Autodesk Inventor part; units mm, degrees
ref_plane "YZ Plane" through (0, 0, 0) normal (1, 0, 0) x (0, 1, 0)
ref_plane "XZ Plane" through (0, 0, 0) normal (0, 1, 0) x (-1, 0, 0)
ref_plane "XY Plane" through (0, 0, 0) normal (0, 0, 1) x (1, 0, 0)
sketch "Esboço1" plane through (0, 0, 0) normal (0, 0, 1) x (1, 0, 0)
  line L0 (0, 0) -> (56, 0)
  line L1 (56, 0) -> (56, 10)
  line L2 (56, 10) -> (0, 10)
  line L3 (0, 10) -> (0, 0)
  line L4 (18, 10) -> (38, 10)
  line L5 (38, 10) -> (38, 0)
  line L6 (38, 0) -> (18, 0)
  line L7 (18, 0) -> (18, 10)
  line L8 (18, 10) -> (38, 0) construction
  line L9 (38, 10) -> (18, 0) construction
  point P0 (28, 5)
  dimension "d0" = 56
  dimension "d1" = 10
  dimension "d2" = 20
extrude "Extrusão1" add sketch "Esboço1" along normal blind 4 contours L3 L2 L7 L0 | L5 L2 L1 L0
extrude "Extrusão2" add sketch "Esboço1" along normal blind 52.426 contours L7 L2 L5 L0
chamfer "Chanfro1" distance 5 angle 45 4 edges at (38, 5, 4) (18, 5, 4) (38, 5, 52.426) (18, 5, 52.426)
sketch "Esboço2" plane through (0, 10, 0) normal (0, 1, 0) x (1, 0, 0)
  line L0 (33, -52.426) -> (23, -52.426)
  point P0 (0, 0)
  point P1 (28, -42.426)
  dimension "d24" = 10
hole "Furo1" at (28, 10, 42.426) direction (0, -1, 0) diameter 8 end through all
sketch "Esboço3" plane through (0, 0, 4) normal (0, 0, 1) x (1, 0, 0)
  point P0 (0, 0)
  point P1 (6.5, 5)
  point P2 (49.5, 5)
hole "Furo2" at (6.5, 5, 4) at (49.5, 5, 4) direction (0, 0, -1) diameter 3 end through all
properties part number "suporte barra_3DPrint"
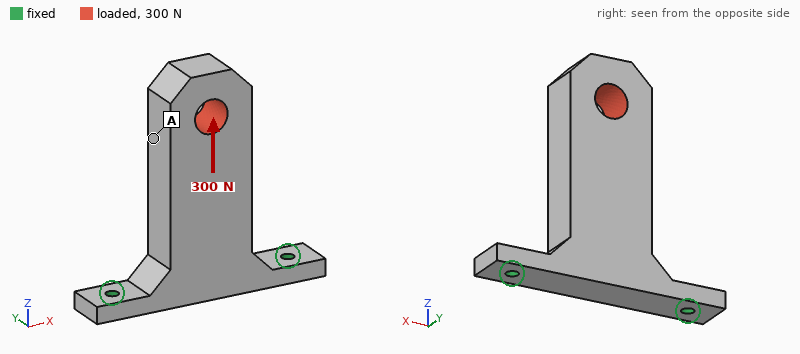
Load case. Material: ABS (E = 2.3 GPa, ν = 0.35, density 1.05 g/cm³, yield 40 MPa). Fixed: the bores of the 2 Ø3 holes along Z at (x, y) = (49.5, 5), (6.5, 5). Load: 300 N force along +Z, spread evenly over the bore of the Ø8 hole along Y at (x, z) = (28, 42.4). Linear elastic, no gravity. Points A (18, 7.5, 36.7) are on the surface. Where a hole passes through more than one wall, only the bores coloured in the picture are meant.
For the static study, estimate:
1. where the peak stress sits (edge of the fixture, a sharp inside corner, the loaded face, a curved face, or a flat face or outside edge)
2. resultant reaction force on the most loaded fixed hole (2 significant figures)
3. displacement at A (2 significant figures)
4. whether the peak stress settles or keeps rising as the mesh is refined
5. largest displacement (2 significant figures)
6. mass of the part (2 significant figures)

edge of the fixture
190 N
0.16 mm
keeps rising
0.18 mm
12 g
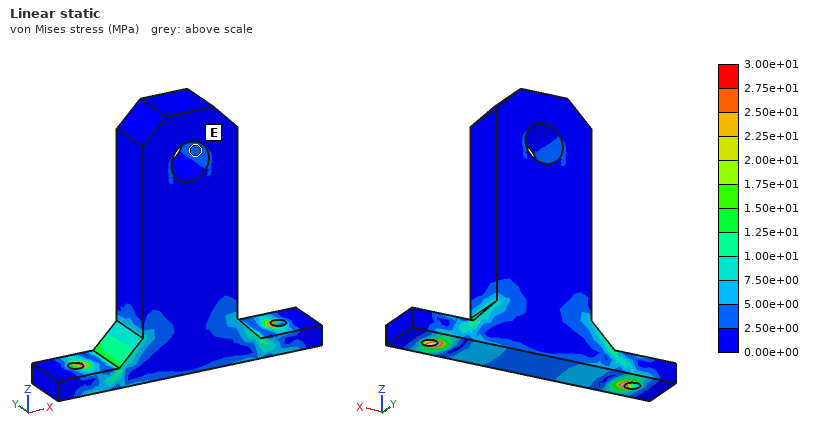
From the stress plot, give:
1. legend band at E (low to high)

2.50e+00 to 5.00e+00 MPa
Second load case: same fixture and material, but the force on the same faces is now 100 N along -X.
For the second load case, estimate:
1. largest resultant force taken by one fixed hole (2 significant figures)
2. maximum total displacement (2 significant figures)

130 N
0.49 mm
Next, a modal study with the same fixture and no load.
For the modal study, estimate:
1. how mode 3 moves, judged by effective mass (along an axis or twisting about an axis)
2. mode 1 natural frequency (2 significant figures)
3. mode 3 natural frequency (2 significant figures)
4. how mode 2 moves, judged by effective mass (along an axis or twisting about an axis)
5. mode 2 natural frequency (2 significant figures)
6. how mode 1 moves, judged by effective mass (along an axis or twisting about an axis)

along Z
330 Hz
2200 Hz
along X
1200 Hz
along Y
